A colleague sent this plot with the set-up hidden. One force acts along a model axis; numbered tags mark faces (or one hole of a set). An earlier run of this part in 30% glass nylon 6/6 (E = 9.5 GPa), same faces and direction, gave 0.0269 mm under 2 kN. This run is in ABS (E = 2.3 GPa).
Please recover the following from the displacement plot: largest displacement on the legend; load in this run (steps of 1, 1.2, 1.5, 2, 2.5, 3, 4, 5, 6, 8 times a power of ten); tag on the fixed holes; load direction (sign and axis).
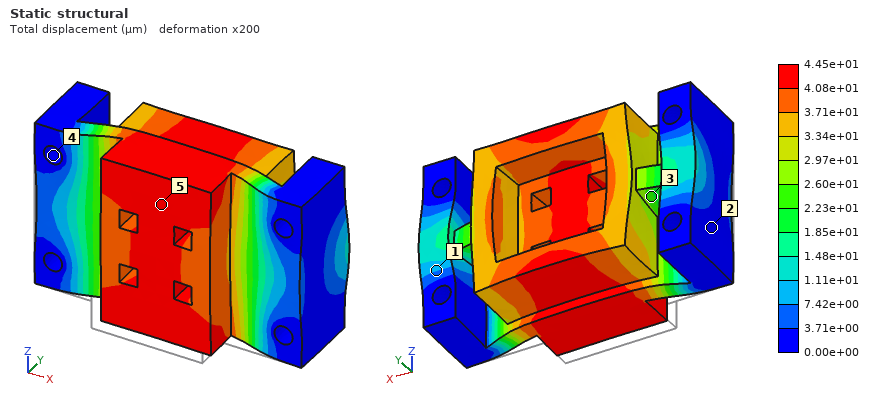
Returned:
4.45e+01 µm
800 N
4
+Y
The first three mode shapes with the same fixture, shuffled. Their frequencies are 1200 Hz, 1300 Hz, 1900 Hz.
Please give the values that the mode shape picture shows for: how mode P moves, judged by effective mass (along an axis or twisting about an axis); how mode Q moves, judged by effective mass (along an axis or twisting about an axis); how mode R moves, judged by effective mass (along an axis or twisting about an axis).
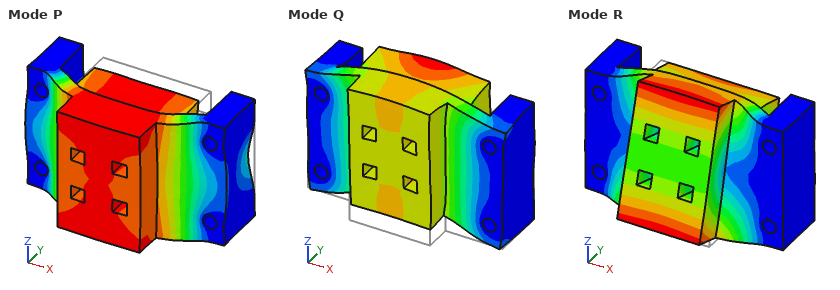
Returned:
along Y
along Z
twisting about X
